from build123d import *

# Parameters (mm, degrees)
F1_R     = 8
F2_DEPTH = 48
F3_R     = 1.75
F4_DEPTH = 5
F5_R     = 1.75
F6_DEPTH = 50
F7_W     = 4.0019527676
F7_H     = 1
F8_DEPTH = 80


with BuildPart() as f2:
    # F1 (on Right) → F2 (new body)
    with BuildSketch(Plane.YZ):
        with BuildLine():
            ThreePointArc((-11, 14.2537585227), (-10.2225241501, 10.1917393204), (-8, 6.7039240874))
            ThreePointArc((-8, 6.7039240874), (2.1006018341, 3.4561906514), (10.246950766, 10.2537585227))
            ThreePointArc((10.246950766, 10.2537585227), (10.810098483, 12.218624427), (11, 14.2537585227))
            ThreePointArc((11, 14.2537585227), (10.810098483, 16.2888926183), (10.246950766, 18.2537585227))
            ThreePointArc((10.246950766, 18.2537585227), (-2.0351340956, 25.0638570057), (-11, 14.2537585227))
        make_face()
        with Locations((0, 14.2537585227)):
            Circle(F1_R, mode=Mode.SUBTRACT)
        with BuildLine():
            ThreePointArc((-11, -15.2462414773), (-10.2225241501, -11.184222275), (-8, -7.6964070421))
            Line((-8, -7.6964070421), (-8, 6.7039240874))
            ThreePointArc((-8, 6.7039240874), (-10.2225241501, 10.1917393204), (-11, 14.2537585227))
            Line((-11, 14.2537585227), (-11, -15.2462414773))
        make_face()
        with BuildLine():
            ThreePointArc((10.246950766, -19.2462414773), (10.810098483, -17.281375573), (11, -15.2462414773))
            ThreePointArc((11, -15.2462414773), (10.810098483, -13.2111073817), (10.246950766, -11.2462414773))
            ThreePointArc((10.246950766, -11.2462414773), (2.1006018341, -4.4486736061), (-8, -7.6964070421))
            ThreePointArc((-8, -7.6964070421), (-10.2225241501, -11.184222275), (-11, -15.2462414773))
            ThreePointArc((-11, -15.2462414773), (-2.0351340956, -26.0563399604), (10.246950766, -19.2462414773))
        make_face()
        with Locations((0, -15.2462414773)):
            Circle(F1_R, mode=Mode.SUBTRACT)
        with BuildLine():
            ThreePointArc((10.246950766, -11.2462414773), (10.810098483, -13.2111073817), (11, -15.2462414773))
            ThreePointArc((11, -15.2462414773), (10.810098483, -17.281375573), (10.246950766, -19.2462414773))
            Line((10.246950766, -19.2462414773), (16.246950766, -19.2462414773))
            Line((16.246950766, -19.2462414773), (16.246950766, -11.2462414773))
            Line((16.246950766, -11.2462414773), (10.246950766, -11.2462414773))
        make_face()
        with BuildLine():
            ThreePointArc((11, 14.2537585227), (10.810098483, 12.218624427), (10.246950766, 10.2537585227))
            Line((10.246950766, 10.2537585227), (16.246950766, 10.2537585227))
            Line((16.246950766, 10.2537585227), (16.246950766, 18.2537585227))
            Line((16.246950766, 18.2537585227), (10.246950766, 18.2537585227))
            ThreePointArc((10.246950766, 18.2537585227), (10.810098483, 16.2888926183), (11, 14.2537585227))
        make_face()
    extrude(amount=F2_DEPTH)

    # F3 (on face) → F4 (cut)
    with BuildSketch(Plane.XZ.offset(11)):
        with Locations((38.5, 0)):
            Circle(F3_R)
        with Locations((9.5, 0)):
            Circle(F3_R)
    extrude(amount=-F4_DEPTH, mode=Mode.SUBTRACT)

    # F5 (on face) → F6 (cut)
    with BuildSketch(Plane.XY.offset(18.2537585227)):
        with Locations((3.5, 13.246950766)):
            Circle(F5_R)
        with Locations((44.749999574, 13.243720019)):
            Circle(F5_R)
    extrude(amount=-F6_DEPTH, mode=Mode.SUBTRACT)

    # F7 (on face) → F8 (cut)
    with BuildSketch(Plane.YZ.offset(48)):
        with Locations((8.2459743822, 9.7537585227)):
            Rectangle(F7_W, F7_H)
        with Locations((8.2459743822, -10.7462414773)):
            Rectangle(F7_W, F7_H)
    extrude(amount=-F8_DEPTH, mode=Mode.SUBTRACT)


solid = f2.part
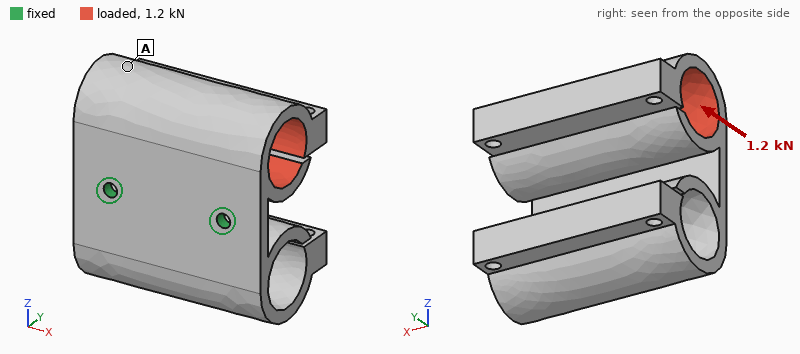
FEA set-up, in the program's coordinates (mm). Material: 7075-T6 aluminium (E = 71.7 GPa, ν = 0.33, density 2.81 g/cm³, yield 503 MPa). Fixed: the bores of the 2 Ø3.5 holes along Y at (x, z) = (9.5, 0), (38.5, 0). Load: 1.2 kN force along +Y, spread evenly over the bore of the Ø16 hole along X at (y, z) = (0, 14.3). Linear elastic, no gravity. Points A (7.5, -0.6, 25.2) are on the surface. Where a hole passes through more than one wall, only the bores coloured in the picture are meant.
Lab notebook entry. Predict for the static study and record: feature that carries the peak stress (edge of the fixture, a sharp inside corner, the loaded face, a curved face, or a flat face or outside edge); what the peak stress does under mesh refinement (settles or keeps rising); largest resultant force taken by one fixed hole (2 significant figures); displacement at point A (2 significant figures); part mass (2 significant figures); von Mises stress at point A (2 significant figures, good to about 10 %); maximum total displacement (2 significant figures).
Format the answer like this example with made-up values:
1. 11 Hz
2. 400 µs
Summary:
1. edge of the fixture
2. keeps rising
3. 600 N
4. 0.36 mm
5. 66 g
6. 26 MPa
7. 0.42 mm
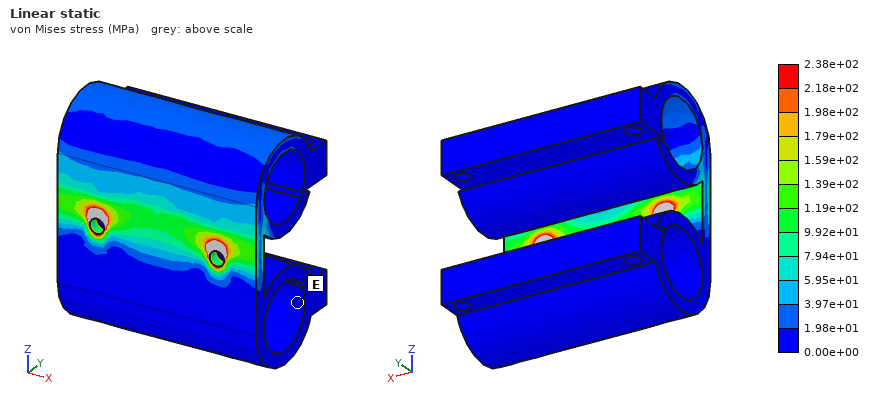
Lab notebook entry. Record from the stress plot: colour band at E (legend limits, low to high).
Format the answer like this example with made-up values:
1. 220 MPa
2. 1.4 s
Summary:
1. 0.00e+00 to 1.98e+01 MPa
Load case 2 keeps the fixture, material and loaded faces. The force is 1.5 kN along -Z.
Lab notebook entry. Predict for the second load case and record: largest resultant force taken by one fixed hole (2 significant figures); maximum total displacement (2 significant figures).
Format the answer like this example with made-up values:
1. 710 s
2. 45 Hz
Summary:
1. 750 N
2. 0.80 mm
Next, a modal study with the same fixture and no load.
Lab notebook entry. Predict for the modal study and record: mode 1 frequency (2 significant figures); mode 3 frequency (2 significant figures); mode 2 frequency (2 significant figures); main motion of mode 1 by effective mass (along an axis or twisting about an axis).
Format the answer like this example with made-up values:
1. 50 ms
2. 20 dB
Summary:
1. 1100 Hz
2. 1900 Hz
3. 1200 Hz
4. along Z
